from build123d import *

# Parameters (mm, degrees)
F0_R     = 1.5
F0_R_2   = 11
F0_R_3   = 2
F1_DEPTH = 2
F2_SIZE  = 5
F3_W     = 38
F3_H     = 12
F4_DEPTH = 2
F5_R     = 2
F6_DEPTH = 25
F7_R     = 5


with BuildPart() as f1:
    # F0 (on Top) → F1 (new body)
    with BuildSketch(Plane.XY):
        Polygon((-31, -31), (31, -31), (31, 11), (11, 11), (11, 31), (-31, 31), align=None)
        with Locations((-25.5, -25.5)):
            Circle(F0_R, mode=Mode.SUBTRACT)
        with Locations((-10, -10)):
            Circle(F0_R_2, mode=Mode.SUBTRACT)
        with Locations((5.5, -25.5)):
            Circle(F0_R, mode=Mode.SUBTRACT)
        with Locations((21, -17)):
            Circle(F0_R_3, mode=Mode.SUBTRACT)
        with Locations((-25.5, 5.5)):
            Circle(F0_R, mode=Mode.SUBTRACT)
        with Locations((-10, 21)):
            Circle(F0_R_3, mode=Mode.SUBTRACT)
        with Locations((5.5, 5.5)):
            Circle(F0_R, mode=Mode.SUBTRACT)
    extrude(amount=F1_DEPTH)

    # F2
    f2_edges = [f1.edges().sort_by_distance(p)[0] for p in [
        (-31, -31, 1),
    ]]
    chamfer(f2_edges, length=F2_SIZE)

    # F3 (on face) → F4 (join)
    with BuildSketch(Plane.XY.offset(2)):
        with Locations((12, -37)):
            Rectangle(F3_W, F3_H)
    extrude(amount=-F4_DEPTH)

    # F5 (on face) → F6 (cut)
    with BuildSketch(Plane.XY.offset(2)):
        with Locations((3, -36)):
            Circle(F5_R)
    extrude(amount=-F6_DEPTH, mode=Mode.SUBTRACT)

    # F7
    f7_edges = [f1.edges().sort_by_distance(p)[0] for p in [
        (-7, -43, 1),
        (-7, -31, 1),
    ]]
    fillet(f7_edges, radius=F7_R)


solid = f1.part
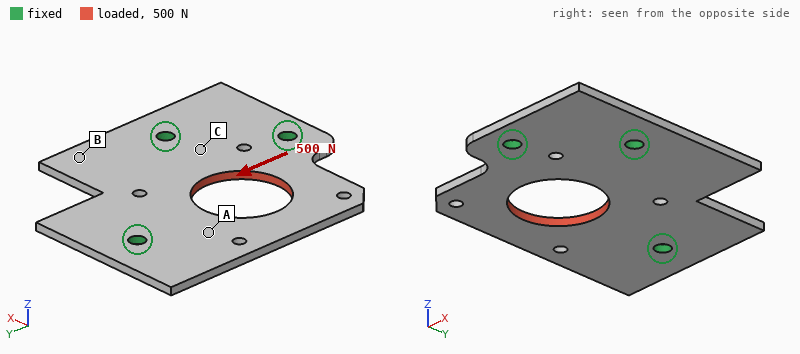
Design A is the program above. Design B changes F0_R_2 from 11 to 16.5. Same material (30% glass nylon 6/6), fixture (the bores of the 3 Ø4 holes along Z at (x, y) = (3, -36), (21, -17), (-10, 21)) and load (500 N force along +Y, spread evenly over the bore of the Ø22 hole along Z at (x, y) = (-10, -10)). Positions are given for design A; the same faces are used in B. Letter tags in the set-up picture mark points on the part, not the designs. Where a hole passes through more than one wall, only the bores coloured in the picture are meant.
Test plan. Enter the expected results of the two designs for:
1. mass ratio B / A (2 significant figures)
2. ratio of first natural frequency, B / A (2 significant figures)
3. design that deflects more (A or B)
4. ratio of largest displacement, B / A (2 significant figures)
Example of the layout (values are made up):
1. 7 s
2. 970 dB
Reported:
1. 0.86
2. 0.99
3. B
4. 2.4
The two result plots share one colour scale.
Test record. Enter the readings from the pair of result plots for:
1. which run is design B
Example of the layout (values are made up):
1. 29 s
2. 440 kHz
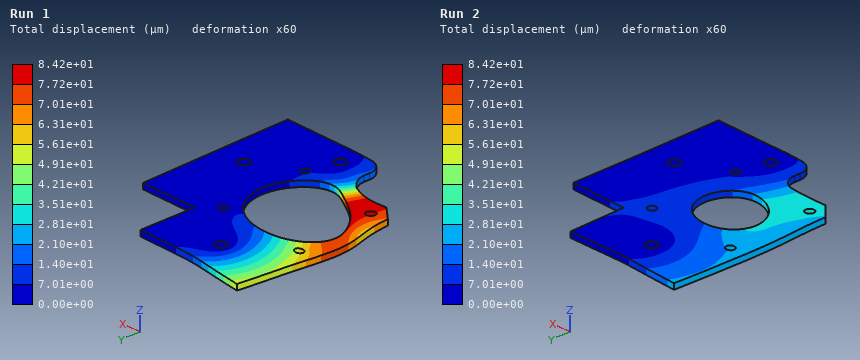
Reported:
1. Run 1
